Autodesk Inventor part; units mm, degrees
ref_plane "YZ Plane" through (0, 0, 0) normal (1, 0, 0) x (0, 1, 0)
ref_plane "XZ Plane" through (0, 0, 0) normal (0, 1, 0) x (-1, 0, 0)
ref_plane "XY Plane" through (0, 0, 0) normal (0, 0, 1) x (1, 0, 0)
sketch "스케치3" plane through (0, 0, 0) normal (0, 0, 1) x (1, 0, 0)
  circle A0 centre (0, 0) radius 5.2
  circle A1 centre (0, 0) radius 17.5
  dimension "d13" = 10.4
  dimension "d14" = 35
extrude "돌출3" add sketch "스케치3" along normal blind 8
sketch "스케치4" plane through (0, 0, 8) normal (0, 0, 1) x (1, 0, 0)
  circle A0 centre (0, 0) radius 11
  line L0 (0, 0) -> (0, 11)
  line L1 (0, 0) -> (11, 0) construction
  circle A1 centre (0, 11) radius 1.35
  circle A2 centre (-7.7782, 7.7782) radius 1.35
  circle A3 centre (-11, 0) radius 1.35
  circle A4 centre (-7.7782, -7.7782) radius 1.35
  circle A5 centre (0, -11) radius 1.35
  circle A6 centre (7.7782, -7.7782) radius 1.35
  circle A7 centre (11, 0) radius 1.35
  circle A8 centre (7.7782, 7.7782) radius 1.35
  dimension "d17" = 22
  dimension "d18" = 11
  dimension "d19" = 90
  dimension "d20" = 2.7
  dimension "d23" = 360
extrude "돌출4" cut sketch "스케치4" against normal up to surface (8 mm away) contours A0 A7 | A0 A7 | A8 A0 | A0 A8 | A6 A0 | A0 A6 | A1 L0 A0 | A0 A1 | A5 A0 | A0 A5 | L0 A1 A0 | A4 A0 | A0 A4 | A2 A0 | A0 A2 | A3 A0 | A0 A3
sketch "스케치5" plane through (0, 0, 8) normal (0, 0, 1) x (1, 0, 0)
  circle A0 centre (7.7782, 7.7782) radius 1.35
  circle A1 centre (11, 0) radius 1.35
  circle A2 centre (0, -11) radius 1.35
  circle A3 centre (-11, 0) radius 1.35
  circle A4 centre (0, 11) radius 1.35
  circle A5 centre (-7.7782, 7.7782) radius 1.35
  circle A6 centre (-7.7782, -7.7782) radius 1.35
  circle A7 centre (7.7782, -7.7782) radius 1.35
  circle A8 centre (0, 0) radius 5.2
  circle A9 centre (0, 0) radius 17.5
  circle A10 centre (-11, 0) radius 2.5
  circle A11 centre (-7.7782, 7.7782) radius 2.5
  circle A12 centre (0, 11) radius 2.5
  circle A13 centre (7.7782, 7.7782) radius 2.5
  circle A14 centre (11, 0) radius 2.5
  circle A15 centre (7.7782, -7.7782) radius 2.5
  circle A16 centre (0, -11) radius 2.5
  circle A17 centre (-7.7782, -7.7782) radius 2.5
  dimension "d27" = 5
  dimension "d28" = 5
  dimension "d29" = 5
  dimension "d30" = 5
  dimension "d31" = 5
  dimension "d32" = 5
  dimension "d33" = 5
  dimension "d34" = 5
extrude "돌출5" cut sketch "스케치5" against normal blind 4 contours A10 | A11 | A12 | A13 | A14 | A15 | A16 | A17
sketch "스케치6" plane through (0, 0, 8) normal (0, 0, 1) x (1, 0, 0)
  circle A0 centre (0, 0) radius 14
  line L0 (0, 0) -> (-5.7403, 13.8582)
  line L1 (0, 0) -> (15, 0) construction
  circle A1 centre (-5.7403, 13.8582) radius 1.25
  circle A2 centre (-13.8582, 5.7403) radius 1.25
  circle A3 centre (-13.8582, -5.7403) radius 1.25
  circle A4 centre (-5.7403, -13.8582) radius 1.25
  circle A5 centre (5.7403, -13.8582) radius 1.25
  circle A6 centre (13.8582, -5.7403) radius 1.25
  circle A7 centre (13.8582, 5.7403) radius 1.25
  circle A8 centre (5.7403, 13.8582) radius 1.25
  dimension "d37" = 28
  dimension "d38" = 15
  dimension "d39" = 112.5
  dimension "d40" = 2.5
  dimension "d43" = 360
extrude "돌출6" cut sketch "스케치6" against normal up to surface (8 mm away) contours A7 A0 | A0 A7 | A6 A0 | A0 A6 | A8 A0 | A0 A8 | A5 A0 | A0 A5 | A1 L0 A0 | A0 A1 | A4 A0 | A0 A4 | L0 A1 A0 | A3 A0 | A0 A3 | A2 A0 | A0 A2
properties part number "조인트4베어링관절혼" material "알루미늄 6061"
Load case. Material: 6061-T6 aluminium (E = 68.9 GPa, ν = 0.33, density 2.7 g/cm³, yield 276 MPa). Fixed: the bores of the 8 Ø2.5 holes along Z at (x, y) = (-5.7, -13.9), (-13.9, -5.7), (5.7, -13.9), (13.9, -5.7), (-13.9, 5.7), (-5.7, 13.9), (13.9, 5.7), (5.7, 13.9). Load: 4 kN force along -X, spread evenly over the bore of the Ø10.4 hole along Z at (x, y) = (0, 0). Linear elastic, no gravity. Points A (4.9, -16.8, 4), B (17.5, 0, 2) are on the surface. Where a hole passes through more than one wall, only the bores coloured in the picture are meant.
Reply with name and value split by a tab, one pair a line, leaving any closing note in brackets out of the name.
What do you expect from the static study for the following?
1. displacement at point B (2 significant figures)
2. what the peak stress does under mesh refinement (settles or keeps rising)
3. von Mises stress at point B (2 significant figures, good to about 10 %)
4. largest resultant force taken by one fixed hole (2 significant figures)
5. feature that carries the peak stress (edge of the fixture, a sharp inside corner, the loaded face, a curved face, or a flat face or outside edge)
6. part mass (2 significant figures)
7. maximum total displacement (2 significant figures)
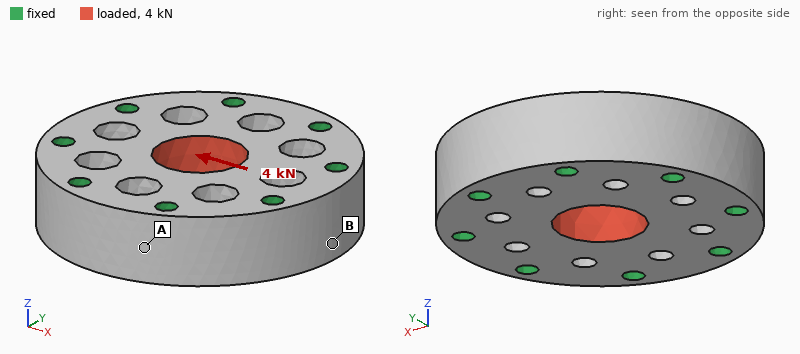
displacement at point B	0.71 µm
what the peak stress does under mesh refinement	keeps rising
von Mises stress at point B	6.6 MPa
largest resultant force taken by one fixed hole	770 N
feature that carries the peak stress	edge of the fixture
part mass	16 g
maximum total displacement	3.0 µm
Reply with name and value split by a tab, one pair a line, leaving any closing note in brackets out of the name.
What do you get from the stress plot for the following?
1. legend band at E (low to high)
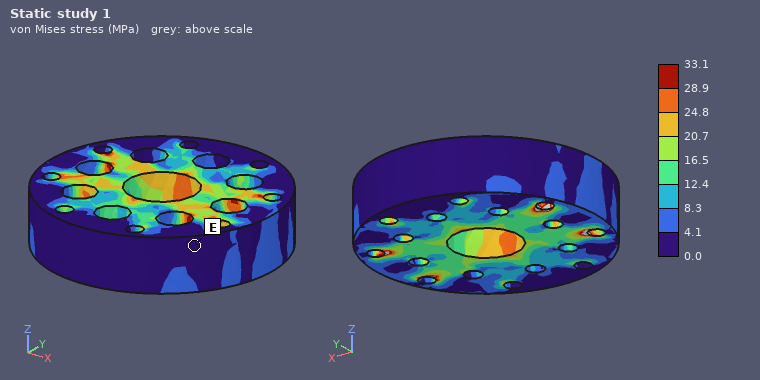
legend band at E	0.0 to 4.1 MPa
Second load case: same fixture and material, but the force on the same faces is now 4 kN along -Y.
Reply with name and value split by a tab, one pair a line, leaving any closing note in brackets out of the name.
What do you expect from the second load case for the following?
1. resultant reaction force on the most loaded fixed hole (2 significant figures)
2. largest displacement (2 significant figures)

resultant reaction force on the most loaded fixed hole	770 N
largest displacement	3.0 µm
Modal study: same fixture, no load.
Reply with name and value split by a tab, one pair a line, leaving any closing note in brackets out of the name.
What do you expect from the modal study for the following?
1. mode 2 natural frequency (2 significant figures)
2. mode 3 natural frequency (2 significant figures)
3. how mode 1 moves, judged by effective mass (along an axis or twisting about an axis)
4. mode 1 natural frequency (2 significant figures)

mode 2 natural frequency	77 kHz
mode 3 natural frequency	77 kHz
how mode 1 moves, judged by effective mass	along Z
mode 1 natural frequency	58 kHz
